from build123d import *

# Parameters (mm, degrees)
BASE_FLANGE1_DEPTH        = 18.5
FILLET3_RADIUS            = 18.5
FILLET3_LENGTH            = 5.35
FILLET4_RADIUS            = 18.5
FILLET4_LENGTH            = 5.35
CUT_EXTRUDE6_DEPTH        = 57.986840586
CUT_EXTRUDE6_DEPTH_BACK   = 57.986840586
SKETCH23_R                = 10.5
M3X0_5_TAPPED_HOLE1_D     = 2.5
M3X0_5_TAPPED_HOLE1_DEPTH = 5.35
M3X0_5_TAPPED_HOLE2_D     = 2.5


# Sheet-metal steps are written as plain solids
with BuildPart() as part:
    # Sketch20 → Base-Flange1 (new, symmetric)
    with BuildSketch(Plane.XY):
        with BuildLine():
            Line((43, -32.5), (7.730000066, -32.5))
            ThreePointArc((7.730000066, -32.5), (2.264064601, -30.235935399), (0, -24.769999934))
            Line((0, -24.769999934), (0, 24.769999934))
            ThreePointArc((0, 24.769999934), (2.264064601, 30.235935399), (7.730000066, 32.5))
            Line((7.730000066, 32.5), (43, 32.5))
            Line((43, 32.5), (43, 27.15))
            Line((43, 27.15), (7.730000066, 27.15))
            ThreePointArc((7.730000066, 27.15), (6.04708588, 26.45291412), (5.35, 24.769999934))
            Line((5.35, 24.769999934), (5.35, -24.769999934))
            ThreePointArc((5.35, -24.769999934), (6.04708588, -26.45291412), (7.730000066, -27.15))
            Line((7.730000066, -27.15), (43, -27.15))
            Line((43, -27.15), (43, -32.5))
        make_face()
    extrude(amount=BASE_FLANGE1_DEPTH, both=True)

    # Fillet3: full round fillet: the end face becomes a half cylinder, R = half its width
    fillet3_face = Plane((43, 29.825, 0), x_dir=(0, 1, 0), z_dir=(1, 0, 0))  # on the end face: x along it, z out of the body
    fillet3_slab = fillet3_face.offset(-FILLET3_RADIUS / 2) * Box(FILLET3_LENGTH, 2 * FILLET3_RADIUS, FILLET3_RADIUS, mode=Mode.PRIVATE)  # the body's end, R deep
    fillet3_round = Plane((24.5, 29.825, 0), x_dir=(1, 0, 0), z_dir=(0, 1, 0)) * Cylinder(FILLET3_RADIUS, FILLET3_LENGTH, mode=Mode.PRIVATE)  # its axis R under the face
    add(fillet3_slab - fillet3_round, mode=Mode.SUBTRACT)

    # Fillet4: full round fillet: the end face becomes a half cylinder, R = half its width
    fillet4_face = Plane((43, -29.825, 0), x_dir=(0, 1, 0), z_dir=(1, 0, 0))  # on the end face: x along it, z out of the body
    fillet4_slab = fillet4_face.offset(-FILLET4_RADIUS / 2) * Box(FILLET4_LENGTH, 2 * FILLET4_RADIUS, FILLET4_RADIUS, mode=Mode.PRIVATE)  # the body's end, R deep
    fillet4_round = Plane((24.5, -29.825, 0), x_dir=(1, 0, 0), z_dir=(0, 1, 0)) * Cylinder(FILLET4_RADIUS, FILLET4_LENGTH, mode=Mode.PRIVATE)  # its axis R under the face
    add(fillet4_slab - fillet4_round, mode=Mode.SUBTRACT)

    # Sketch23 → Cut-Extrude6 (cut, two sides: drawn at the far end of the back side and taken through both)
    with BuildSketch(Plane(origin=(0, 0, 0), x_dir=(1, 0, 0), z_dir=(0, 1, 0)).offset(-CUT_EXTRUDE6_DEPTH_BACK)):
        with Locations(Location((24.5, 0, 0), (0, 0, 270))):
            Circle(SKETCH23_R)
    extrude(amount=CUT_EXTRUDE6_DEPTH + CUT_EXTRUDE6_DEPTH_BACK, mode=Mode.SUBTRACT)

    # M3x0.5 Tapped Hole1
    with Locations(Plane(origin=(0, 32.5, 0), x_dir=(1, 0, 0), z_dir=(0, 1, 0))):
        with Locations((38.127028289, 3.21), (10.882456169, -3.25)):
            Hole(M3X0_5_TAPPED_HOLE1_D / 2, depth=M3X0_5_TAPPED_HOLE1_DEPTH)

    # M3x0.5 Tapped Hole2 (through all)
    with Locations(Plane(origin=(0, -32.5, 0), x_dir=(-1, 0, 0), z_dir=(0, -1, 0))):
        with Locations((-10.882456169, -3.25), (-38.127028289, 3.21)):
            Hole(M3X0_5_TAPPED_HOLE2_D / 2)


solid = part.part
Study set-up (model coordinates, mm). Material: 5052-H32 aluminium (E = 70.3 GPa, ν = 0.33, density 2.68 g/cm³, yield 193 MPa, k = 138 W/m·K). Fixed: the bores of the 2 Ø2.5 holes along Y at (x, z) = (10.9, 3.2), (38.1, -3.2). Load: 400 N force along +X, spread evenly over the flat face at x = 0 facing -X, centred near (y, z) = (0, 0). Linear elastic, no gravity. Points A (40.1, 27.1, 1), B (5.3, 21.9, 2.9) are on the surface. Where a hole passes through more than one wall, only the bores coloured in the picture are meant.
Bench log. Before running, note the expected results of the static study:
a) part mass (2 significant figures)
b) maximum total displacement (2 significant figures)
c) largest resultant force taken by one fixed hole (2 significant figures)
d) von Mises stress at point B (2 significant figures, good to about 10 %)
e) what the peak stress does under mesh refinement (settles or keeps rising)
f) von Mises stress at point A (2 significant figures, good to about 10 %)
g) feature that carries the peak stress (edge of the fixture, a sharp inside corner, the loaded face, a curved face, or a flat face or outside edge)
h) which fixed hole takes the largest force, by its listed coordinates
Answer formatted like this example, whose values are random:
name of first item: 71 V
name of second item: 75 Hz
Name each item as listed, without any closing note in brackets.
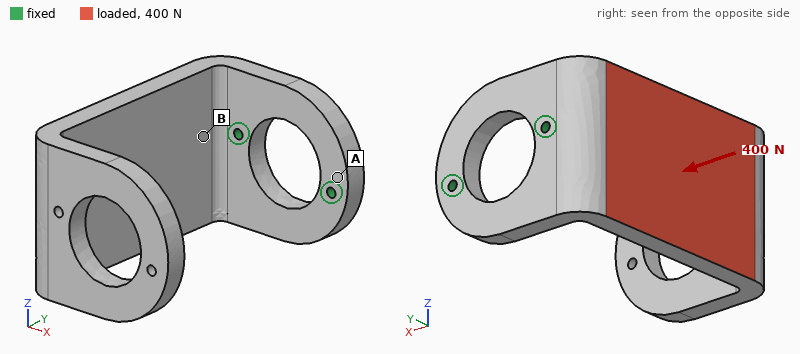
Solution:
part mass: 58 g
maximum total displacement: 0.67 mm
largest resultant force taken by one fixed hole: 410 N
von Mises stress at point B: 43 MPa
what the peak stress does under mesh refinement: keeps rising
von Mises stress at point A: 17 MPa
feature that carries the peak stress: edge of the fixture
which fixed hole takes the largest force, by its listed coordinates: (10.9, 3.2)
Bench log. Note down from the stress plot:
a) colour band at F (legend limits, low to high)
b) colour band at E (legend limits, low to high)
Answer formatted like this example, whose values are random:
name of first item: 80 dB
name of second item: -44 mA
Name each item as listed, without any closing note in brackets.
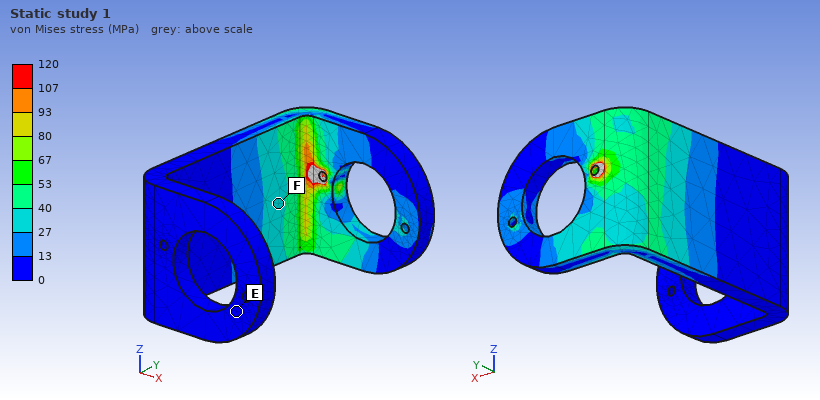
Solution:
colour band at F: 27 to 40 MPa
colour band at E: 0 to 13 MPa
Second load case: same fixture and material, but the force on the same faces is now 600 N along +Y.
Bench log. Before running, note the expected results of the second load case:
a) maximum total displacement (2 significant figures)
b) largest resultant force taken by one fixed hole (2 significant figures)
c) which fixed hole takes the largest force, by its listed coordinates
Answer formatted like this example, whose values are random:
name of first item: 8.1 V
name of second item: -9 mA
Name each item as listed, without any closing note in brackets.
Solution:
maximum total displacement: 0.22 mm
largest resultant force taken by one fixed hole: 670 N
which fixed hole takes the largest force, by its listed coordinates: (10.9, 3.2)
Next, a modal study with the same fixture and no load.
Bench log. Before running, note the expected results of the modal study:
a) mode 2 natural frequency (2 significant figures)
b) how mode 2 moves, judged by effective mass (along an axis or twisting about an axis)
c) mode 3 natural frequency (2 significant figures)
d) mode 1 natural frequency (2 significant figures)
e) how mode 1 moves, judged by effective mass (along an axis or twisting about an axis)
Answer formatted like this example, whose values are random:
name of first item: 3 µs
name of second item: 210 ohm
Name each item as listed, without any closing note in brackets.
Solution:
mode 2 natural frequency: 830 Hz
how mode 2 moves, judged by effective mass: along Z
mode 3 natural frequency: 2000 Hz
mode 1 natural frequency: 570 Hz
how mode 1 moves, judged by effective mass: along X
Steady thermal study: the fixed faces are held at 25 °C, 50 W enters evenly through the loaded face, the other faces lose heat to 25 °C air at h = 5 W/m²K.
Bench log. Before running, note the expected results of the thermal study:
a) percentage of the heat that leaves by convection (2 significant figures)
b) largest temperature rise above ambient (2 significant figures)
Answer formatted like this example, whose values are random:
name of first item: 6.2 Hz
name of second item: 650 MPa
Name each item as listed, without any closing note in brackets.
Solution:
percentage of the heat that leaves by convection: 4.3 %
largest temperature rise above ambient: 77 K
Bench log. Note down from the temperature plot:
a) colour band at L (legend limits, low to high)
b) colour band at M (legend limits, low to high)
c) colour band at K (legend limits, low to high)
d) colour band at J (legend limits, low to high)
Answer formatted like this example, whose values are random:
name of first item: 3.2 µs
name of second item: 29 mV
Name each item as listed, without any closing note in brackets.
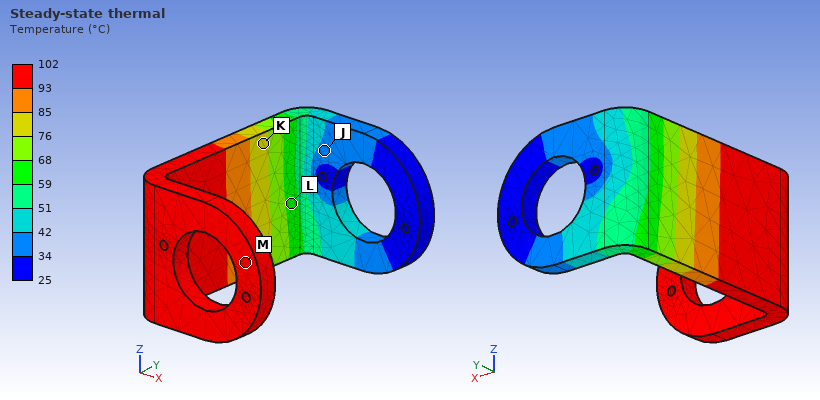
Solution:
colour band at L: 59 to 68 °C
colour band at M: 93 to 102 °C
colour band at K: 76 to 85 °C
colour band at J: 34 to 42 °C
